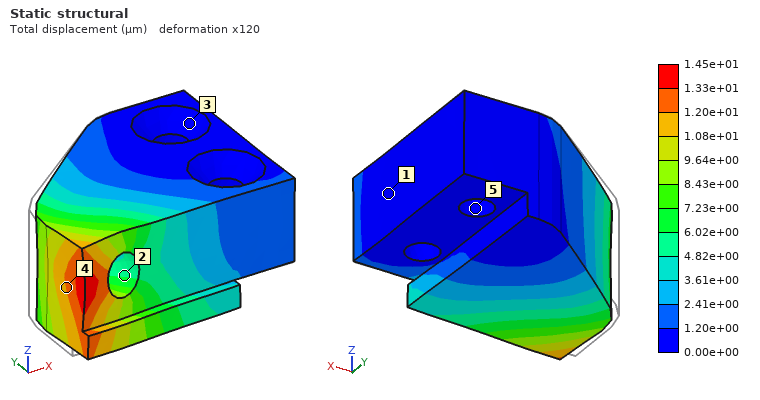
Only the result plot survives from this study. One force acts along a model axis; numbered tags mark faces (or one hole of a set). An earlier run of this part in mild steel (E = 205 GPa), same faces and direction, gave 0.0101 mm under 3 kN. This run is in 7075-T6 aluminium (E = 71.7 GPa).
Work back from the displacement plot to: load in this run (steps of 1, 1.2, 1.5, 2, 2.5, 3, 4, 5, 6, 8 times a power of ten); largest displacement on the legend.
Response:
1.5 kN
1.45e+01 µm
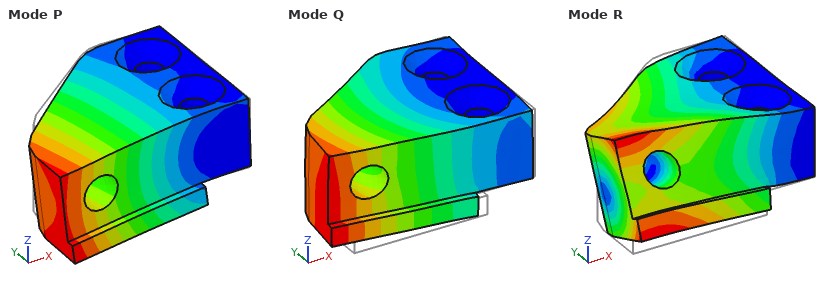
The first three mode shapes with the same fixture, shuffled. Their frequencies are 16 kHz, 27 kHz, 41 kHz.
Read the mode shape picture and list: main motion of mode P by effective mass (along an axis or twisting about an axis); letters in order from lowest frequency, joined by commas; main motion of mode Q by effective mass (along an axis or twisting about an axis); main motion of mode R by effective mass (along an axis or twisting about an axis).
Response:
along Z
P, Q, R
along Y
twisting about X
